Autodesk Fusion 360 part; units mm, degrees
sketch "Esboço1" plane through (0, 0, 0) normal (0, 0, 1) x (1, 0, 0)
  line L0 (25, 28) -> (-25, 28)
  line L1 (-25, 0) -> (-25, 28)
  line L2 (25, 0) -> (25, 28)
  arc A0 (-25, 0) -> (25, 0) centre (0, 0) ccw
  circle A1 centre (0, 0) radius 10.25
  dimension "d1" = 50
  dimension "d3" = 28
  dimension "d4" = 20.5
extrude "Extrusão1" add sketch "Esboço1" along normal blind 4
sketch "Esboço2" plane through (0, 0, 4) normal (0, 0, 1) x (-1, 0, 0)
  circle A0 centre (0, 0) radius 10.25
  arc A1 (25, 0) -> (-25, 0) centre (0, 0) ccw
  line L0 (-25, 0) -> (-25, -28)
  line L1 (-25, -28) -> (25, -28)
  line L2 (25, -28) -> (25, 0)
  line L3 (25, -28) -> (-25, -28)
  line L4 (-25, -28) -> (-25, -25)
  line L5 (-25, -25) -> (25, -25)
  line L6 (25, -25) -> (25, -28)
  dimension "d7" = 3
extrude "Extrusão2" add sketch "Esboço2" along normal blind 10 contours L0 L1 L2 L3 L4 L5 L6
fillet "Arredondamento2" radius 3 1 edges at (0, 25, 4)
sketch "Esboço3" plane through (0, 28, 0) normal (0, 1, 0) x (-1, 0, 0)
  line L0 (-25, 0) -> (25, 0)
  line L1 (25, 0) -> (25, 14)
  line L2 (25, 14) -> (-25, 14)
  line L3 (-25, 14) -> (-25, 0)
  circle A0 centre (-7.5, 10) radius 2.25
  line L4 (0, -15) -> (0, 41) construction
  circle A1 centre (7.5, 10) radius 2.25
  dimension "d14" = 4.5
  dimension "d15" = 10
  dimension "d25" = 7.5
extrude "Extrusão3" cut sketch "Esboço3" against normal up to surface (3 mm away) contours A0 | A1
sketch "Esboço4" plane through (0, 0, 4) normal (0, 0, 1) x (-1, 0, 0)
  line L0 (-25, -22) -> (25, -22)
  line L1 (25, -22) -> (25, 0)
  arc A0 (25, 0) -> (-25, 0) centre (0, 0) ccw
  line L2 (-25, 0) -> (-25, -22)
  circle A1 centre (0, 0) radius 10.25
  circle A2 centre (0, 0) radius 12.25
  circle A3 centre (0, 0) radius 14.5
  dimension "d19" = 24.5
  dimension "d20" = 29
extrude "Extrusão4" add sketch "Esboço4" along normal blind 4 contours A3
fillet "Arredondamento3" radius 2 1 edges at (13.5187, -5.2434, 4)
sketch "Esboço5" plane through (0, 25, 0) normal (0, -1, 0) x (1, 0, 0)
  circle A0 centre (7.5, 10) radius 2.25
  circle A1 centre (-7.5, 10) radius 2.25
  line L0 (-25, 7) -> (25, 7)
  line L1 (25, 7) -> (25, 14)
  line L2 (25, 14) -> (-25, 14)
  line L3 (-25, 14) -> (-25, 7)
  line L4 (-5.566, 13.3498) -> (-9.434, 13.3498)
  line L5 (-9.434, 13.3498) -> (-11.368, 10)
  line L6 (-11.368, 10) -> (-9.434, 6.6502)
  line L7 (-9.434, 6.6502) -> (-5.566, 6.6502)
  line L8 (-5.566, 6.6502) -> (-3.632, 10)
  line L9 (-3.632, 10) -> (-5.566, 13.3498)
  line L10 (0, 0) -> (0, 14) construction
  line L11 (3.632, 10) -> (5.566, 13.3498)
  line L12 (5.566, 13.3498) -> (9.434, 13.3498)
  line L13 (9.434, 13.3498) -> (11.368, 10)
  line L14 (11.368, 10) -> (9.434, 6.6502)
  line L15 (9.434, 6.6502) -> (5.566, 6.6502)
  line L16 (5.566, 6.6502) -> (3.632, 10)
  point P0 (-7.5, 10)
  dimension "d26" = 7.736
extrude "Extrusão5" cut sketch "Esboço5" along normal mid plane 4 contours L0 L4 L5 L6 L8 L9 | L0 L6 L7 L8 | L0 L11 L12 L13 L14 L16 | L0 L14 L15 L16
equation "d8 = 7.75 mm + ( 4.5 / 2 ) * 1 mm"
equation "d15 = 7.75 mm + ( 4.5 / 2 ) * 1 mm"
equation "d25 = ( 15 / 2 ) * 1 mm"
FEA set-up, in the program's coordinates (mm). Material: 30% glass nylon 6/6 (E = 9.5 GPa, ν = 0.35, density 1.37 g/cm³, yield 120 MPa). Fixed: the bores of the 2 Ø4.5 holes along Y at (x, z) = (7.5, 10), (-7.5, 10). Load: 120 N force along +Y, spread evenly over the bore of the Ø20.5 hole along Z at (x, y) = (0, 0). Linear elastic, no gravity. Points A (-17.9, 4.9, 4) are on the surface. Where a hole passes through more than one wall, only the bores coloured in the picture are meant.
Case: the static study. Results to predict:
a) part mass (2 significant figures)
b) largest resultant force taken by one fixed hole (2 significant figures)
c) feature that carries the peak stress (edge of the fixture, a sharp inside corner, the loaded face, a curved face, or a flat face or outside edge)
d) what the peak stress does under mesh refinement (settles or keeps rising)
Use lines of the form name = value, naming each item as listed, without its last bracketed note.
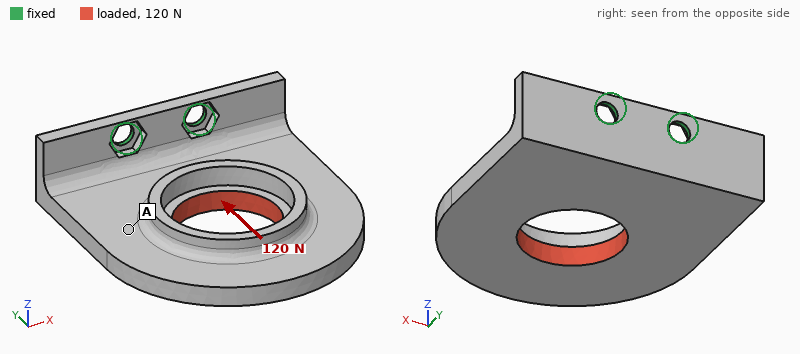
part mass = 14 g
largest resultant force taken by one fixed hole = 60 N
feature that carries the peak stress = edge of the fixture
what the peak stress does under mesh refinement = keeps rising
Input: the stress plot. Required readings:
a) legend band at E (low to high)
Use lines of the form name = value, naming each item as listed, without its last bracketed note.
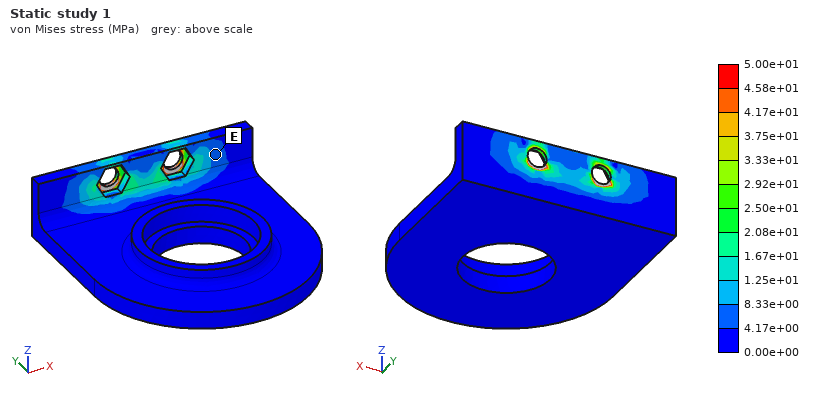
legend band at E = 4.17e+00 to 8.33e+00 MPa
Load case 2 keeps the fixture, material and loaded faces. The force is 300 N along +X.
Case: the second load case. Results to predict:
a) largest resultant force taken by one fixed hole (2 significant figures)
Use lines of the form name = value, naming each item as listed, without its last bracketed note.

largest resultant force taken by one fixed hole = 550 N
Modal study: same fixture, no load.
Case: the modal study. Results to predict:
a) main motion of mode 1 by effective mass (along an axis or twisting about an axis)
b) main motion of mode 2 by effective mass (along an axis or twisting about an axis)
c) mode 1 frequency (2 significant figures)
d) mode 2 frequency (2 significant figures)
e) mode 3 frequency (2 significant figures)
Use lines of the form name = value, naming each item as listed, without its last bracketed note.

main motion of mode 1 by effective mass = along Z
main motion of mode 2 by effective mass = along X
mode 1 frequency = 370 Hz
mode 2 frequency = 970 Hz
mode 3 frequency = 1800 Hz
